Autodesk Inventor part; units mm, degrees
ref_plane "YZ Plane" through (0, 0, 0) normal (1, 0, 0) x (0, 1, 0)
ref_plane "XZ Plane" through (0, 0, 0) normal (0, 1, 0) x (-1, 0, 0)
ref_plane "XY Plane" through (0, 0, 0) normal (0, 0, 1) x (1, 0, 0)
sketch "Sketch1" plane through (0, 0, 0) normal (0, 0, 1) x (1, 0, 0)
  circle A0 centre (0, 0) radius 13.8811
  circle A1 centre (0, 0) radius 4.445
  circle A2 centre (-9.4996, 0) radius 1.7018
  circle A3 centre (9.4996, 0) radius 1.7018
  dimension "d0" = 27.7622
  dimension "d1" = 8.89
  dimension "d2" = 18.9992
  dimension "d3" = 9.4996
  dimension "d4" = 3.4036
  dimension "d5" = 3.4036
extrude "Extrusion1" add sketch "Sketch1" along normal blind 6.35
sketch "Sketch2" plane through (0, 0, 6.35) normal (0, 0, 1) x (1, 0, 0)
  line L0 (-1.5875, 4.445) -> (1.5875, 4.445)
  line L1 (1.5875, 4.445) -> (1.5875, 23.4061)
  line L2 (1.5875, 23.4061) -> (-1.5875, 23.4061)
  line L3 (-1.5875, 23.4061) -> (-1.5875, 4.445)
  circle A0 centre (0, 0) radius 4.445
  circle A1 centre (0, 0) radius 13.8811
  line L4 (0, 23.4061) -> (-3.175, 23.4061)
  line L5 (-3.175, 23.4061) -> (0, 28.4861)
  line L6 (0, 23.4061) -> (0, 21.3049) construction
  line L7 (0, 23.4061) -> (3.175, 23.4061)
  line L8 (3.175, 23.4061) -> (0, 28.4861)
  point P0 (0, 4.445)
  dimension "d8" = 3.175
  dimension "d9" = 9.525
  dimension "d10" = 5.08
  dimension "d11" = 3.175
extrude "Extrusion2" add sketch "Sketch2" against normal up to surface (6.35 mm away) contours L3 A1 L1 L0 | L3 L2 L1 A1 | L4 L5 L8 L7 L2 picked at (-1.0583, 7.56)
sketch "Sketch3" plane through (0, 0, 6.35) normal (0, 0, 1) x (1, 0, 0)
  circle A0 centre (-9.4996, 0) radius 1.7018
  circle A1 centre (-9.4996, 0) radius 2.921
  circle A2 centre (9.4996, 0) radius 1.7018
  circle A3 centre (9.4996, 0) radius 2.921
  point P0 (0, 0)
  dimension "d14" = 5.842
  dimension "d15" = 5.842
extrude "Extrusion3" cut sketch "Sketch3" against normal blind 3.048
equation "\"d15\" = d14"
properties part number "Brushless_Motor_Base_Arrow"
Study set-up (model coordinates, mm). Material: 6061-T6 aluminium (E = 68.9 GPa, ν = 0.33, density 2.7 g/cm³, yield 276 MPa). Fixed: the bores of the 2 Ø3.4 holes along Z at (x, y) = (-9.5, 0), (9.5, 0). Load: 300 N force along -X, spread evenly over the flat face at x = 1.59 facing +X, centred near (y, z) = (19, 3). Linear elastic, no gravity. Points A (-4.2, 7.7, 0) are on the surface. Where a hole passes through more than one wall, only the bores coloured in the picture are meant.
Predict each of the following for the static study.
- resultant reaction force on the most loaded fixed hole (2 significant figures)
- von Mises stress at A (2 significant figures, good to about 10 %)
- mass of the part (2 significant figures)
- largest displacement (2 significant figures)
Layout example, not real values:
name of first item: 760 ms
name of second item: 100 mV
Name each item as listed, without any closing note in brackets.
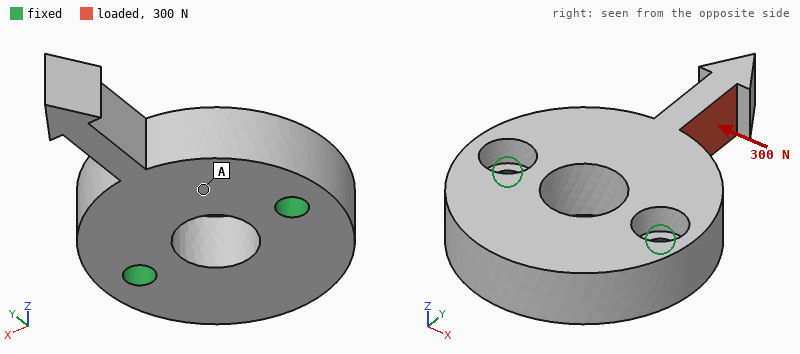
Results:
resultant reaction force on the most loaded fixed hole: 310 N
von Mises stress at A: 10 MPa
mass of the part: 9.5 g
largest displacement: 77 µm
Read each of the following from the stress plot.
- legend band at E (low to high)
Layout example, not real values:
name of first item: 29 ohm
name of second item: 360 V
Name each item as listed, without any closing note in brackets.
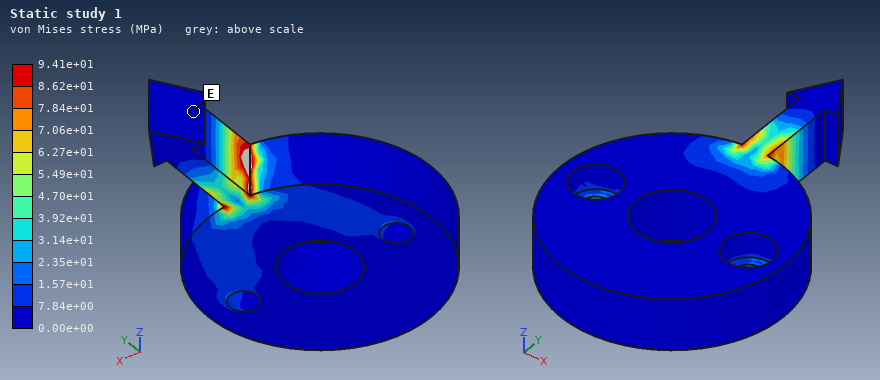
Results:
legend band at E: 0.00e+00 to 7.84e+00 MPa
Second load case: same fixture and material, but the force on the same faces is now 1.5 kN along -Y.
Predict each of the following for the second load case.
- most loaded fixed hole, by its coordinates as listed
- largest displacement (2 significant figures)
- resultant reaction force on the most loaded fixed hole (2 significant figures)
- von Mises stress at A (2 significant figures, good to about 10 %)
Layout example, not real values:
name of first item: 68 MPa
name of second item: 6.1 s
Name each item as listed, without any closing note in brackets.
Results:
most loaded fixed hole, by its coordinates as listed: (9.5, 0)
largest displacement: 0.15 mm
resultant reaction force on the most loaded fixed hole: 930 N
von Mises stress at A: 21 MPa
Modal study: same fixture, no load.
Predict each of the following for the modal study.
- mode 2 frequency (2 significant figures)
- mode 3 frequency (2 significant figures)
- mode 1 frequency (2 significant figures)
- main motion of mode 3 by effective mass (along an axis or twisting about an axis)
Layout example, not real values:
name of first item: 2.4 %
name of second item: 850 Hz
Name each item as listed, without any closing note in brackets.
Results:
mode 2 frequency: 11 kHz
mode 3 frequency: 17 kHz
mode 1 frequency: 8500 Hz
main motion of mode 3 by effective mass: along Z
